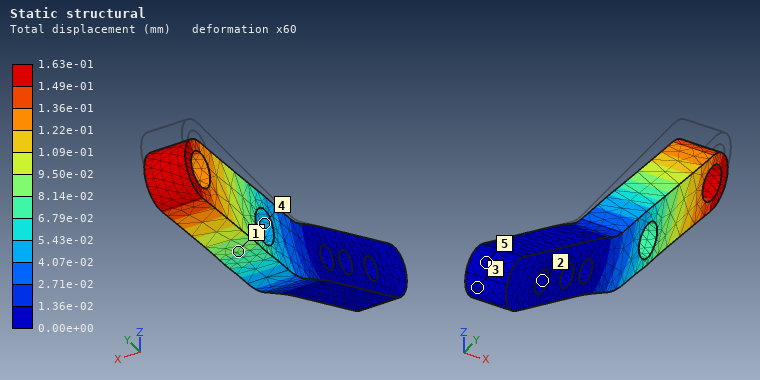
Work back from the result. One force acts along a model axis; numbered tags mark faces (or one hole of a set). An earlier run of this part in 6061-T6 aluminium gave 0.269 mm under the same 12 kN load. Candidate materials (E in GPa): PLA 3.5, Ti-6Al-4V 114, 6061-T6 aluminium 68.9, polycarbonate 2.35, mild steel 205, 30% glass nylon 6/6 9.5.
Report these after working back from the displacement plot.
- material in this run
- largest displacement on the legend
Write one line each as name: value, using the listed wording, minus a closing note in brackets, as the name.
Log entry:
material in this run: Ti-6Al-4V
largest displacement on the legend: 1.63e-01 mm
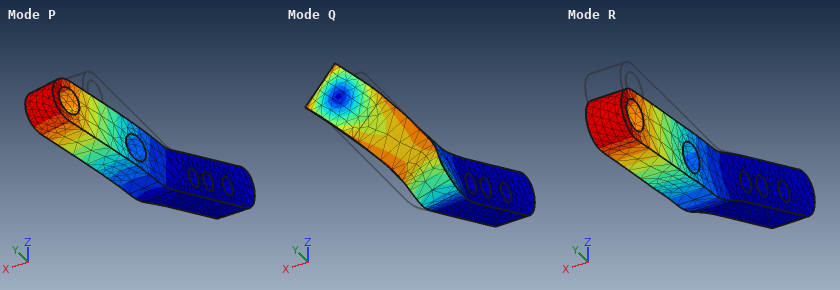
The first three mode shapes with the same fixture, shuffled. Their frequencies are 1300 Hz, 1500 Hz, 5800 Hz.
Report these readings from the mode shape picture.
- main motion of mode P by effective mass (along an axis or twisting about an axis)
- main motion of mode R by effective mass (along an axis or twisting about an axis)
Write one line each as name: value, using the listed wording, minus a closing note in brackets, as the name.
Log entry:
main motion of mode P by effective mass: along X
main motion of mode R by effective mass: along Z
